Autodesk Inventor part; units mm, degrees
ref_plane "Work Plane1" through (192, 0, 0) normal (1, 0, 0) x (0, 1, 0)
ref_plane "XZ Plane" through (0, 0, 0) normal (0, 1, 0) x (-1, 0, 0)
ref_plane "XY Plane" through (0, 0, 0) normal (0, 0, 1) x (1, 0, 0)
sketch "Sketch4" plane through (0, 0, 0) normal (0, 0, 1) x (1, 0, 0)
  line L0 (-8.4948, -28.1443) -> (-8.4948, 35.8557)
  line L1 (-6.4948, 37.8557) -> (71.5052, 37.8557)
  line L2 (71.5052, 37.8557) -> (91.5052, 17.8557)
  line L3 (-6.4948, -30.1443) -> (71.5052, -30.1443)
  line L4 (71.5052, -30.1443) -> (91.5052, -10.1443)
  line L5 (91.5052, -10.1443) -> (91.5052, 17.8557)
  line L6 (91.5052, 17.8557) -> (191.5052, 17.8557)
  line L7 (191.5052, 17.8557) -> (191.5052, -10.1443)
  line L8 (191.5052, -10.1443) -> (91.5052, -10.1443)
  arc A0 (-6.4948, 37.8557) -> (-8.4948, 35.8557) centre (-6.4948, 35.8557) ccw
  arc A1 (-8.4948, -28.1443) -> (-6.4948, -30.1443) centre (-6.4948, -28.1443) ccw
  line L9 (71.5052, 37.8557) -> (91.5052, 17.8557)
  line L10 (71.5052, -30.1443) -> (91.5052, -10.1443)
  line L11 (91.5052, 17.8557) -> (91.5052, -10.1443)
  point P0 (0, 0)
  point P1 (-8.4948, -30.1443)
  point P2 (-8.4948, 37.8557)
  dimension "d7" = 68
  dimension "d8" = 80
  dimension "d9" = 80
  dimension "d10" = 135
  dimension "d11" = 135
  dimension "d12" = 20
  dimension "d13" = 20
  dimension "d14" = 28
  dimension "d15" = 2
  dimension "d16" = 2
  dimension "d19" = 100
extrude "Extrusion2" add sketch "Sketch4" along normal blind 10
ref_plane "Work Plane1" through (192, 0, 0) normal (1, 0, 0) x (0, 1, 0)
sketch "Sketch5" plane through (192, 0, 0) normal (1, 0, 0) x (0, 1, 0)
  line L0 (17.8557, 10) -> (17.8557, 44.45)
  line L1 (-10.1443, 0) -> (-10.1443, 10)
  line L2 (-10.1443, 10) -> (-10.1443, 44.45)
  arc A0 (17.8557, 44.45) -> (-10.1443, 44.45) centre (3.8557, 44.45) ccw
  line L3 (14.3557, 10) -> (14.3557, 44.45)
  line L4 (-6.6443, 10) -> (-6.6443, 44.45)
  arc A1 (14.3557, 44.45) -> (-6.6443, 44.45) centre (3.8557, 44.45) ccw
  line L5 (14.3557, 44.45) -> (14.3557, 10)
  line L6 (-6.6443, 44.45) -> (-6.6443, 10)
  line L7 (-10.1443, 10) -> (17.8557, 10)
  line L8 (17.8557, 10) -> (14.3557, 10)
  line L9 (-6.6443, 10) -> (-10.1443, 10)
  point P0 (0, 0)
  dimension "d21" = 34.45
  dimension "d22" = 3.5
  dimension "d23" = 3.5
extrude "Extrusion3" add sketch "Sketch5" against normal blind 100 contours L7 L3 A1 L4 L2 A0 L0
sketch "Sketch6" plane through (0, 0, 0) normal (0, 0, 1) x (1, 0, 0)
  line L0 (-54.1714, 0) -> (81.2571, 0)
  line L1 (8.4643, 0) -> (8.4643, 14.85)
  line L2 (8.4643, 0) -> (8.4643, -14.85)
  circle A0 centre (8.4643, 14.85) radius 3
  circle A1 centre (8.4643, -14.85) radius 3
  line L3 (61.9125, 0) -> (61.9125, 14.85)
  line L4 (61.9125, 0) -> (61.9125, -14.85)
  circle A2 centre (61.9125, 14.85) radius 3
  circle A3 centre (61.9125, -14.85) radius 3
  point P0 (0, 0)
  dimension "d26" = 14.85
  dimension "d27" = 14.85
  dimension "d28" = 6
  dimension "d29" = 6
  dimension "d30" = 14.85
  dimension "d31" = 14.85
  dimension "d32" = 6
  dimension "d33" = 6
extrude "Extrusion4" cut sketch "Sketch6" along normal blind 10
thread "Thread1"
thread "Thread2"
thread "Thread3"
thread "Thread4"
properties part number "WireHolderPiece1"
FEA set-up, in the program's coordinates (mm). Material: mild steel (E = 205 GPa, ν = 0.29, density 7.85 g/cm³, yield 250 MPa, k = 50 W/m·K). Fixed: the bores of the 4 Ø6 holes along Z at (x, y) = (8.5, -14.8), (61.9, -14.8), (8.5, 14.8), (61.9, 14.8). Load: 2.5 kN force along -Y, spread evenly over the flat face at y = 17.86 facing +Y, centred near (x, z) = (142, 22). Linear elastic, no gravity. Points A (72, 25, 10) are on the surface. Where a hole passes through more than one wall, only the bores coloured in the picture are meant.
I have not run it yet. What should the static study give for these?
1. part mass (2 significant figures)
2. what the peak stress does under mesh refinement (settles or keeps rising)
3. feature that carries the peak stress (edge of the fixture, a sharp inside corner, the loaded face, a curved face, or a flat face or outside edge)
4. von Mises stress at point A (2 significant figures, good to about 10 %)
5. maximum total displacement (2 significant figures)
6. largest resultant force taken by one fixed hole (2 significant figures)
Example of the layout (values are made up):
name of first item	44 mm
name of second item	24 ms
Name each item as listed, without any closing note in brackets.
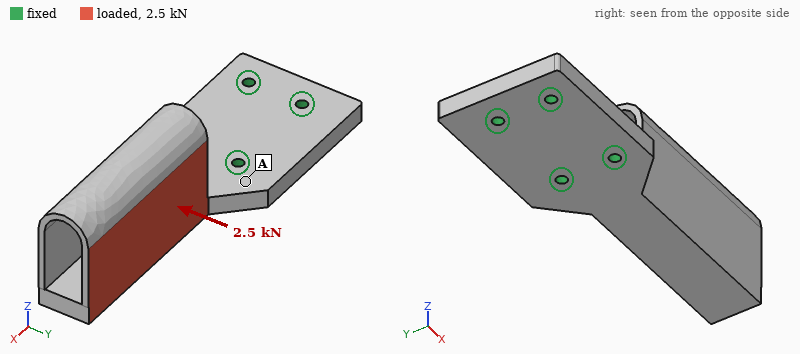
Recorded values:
part mass	1.0 kg
what the peak stress does under mesh refinement	keeps rising
feature that carries the peak stress	a sharp inside corner
von Mises stress at point A	15 MPa
maximum total displacement	0.21 mm
largest resultant force taken by one fixed hole	5.0 kN
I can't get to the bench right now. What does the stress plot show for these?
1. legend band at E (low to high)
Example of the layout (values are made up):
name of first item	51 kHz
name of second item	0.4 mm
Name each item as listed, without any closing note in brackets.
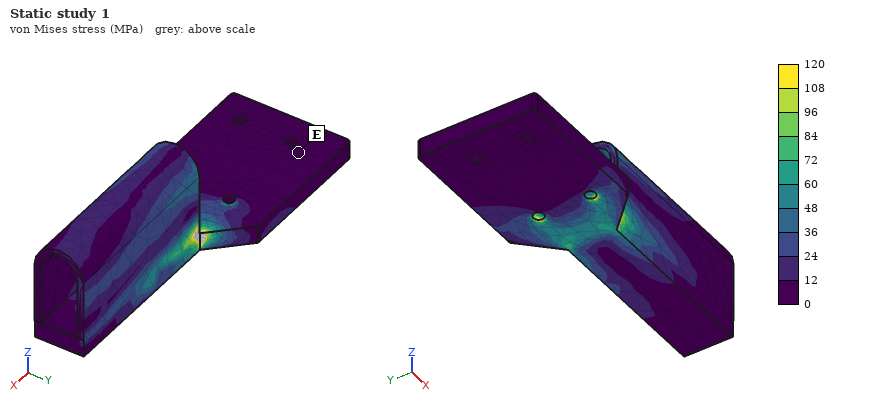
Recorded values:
legend band at E	0 to 12 MPa
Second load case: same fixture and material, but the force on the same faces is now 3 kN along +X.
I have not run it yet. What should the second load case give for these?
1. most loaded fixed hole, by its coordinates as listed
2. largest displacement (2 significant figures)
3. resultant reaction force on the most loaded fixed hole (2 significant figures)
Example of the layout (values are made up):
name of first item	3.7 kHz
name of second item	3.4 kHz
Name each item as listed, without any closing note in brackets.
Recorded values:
most loaded fixed hole, by its coordinates as listed	(61.9, 14.8)
largest displacement	0.39 mm
resultant reaction force on the most loaded fixed hole	2.5 kN
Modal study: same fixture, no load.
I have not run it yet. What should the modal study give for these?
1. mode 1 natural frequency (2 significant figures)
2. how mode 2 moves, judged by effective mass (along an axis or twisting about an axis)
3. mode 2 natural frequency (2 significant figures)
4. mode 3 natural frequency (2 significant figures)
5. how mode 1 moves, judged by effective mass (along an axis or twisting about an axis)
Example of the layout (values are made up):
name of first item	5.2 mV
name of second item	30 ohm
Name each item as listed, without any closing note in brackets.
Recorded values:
mode 1 natural frequency	400 Hz
how mode 2 moves, judged by effective mass	along Y
mode 2 natural frequency	950 Hz
mode 3 natural frequency	1600 Hz
how mode 1 moves, judged by effective mass	along Z
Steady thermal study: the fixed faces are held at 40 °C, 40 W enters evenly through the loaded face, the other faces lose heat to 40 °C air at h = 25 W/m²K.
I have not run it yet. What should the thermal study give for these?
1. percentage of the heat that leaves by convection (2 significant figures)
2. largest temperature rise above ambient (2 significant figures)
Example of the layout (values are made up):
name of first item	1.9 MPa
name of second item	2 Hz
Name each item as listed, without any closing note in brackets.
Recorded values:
percentage of the heat that leaves by convection	67 %
largest temperature rise above ambient	60 K
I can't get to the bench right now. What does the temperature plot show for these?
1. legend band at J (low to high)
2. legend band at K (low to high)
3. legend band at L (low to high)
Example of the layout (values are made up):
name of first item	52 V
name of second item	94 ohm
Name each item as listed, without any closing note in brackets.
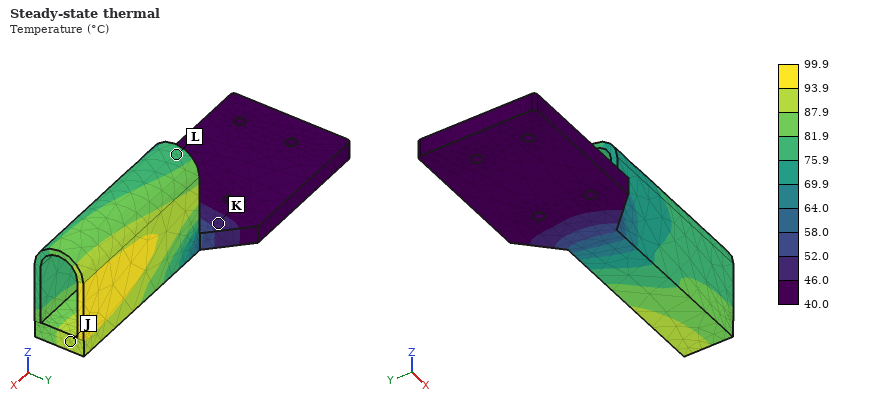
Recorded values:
legend band at J	87.9 to 93.9 °C
legend band at K	46.0 to 52.0 °C
legend band at L	75.9 to 81.9 °C
